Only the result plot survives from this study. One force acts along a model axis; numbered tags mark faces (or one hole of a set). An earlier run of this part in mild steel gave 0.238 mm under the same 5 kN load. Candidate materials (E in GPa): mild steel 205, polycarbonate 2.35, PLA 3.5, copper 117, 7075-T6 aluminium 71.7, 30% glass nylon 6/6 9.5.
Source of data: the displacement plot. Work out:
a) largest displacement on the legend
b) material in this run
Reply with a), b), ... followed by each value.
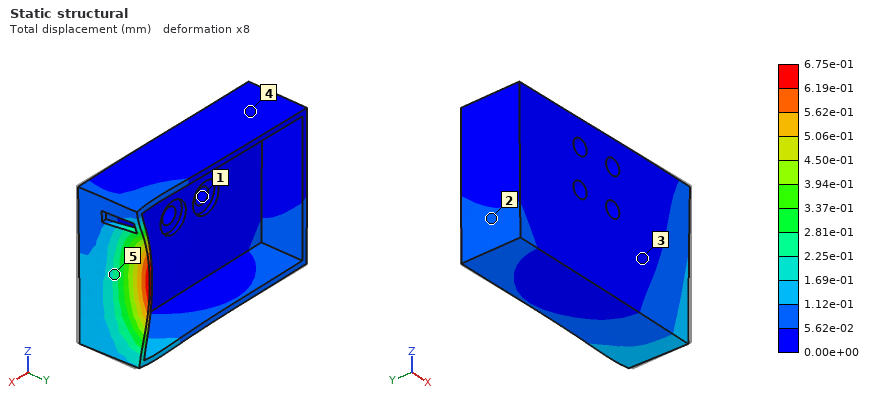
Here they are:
a) 6.75e-01 mm
b) 7075-T6 aluminium
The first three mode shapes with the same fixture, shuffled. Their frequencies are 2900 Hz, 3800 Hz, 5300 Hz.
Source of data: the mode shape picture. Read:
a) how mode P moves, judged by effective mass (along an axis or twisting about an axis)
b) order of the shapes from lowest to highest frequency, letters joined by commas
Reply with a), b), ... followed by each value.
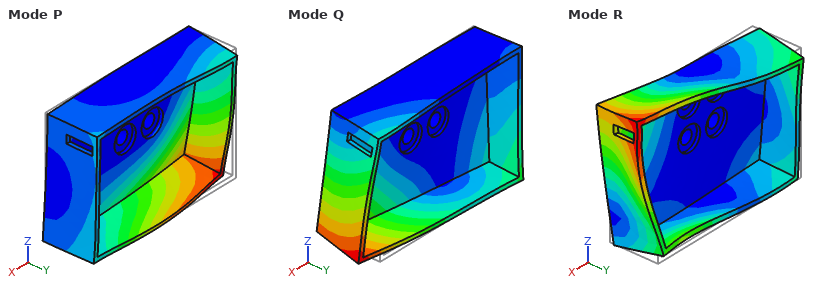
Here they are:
a) along Y
b) Q, P, R
